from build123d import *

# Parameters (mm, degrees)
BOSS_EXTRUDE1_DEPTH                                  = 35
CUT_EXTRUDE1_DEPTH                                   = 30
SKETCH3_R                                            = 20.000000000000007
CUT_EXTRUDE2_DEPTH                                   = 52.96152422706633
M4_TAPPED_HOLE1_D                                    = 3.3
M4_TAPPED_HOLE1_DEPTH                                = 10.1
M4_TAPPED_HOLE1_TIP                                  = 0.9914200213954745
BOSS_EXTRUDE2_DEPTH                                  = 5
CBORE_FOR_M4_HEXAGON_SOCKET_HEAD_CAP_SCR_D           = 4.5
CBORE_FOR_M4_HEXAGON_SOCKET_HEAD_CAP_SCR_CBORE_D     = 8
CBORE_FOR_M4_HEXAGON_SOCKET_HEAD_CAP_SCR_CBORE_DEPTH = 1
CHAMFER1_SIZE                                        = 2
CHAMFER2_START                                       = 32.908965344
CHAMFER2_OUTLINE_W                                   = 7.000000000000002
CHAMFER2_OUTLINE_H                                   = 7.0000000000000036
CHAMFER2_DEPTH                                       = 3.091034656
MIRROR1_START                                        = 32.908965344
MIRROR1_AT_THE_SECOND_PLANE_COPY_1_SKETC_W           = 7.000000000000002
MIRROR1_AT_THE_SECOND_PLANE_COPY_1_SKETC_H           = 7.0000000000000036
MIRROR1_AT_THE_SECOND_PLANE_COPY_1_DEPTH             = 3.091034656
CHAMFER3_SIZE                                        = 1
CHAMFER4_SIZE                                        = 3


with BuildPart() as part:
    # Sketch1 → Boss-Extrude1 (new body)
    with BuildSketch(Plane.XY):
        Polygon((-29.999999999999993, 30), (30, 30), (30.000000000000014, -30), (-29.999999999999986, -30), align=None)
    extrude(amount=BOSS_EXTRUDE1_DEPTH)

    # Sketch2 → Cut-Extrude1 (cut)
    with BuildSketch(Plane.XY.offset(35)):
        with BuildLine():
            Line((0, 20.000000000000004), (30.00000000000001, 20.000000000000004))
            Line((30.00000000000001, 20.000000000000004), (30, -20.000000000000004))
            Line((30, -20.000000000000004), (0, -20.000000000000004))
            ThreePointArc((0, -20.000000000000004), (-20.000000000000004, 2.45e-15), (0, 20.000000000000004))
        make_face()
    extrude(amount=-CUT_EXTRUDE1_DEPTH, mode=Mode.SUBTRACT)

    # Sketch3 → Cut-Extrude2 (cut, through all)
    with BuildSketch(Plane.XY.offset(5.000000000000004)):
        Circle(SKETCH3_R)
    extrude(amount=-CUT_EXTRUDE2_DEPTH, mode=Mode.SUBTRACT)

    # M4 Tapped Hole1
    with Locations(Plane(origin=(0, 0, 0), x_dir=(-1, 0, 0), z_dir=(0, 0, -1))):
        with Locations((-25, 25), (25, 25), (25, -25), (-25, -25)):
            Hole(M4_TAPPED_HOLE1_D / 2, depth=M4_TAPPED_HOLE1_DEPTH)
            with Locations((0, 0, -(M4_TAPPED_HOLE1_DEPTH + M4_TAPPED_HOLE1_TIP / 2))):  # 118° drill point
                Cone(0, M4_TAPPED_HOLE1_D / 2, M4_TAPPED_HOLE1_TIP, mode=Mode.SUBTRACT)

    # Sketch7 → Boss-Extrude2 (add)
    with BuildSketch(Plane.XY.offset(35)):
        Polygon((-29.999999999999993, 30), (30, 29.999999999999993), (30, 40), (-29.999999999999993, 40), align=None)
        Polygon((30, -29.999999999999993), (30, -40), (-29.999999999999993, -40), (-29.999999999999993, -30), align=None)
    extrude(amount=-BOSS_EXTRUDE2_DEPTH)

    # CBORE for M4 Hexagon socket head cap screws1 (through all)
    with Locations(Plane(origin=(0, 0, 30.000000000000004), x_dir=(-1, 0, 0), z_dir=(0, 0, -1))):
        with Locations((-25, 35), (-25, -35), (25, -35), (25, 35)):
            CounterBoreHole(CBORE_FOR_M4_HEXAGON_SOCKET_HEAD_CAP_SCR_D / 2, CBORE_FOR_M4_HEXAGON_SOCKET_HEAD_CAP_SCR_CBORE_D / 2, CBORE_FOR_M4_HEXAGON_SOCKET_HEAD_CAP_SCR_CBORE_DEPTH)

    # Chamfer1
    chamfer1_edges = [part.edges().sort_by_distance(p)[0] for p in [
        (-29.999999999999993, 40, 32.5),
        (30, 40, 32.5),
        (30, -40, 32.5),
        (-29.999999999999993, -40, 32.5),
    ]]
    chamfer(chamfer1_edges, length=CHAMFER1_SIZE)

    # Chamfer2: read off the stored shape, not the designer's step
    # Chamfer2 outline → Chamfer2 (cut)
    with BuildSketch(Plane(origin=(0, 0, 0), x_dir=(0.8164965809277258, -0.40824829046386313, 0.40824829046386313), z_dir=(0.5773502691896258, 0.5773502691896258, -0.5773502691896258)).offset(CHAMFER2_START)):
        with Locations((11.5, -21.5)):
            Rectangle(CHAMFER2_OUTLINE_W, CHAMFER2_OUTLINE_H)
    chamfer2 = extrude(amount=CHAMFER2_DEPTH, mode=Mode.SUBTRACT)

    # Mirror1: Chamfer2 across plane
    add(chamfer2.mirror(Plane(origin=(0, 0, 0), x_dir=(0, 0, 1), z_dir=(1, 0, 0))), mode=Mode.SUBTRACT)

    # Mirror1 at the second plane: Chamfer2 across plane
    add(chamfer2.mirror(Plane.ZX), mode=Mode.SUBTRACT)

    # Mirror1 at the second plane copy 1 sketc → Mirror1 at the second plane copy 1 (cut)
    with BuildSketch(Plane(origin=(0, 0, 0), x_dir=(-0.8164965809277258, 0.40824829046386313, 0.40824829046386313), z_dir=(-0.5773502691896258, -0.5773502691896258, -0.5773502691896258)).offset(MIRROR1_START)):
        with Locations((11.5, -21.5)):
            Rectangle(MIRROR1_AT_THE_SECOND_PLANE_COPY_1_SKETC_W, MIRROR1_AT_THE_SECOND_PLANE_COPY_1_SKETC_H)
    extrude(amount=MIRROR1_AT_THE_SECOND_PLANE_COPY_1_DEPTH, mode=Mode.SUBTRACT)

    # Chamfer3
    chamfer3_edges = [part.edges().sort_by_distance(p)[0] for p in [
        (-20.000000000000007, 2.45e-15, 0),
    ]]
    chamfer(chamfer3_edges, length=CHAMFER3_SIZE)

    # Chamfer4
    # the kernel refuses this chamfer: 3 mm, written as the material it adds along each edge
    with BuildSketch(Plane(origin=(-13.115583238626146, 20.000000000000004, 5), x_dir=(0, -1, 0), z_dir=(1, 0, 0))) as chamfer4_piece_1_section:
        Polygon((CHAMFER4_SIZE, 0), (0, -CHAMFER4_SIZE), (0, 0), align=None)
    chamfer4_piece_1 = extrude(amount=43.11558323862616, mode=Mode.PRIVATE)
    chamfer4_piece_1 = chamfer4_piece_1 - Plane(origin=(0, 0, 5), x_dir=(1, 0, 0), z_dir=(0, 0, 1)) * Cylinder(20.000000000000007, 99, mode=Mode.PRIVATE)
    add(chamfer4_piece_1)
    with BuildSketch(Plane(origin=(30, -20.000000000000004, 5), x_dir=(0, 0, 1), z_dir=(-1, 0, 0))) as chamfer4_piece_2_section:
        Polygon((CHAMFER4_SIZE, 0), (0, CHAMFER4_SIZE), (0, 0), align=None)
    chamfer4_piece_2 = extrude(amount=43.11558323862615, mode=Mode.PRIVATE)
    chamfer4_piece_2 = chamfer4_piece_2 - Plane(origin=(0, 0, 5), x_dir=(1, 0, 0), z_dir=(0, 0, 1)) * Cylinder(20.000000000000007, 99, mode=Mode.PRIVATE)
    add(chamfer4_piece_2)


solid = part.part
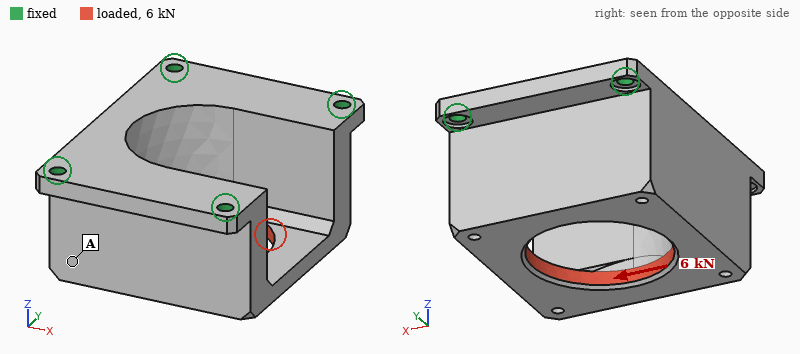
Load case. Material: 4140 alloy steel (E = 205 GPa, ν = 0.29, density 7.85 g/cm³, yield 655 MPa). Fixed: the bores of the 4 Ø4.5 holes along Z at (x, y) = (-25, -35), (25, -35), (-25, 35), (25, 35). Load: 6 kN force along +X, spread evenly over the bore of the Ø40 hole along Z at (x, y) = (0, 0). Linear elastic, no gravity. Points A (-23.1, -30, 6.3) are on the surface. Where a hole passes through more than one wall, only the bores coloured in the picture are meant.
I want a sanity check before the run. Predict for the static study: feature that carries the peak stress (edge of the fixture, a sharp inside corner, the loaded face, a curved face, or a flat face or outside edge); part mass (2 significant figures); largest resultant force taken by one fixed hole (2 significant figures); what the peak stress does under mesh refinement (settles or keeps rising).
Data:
edge of the fixture
550 g
2.6 kN
keeps rising
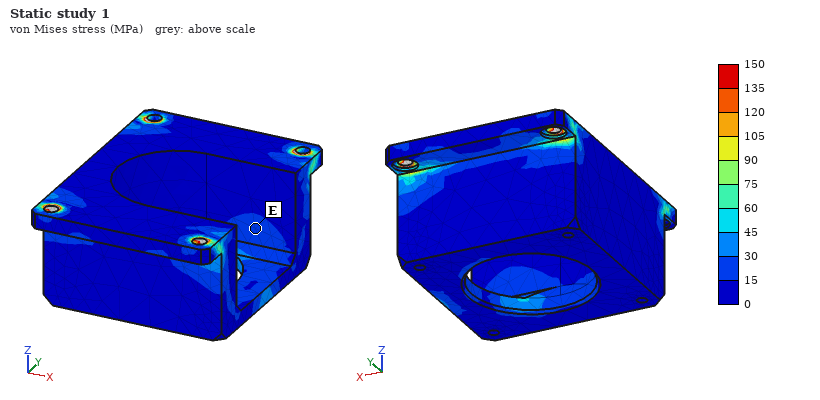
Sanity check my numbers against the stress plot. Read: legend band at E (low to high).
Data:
15 to 30 MPa
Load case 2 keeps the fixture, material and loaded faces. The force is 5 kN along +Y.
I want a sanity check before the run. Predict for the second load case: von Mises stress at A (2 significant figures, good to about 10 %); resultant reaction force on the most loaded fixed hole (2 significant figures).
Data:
13 MPa
2.8 kN
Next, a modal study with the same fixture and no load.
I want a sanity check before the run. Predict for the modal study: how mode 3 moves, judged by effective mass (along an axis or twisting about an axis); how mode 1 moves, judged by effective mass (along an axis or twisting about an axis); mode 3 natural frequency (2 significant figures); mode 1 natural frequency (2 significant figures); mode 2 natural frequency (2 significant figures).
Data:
along Z
along Y
7800 Hz
5200 Hz
6500 Hz
